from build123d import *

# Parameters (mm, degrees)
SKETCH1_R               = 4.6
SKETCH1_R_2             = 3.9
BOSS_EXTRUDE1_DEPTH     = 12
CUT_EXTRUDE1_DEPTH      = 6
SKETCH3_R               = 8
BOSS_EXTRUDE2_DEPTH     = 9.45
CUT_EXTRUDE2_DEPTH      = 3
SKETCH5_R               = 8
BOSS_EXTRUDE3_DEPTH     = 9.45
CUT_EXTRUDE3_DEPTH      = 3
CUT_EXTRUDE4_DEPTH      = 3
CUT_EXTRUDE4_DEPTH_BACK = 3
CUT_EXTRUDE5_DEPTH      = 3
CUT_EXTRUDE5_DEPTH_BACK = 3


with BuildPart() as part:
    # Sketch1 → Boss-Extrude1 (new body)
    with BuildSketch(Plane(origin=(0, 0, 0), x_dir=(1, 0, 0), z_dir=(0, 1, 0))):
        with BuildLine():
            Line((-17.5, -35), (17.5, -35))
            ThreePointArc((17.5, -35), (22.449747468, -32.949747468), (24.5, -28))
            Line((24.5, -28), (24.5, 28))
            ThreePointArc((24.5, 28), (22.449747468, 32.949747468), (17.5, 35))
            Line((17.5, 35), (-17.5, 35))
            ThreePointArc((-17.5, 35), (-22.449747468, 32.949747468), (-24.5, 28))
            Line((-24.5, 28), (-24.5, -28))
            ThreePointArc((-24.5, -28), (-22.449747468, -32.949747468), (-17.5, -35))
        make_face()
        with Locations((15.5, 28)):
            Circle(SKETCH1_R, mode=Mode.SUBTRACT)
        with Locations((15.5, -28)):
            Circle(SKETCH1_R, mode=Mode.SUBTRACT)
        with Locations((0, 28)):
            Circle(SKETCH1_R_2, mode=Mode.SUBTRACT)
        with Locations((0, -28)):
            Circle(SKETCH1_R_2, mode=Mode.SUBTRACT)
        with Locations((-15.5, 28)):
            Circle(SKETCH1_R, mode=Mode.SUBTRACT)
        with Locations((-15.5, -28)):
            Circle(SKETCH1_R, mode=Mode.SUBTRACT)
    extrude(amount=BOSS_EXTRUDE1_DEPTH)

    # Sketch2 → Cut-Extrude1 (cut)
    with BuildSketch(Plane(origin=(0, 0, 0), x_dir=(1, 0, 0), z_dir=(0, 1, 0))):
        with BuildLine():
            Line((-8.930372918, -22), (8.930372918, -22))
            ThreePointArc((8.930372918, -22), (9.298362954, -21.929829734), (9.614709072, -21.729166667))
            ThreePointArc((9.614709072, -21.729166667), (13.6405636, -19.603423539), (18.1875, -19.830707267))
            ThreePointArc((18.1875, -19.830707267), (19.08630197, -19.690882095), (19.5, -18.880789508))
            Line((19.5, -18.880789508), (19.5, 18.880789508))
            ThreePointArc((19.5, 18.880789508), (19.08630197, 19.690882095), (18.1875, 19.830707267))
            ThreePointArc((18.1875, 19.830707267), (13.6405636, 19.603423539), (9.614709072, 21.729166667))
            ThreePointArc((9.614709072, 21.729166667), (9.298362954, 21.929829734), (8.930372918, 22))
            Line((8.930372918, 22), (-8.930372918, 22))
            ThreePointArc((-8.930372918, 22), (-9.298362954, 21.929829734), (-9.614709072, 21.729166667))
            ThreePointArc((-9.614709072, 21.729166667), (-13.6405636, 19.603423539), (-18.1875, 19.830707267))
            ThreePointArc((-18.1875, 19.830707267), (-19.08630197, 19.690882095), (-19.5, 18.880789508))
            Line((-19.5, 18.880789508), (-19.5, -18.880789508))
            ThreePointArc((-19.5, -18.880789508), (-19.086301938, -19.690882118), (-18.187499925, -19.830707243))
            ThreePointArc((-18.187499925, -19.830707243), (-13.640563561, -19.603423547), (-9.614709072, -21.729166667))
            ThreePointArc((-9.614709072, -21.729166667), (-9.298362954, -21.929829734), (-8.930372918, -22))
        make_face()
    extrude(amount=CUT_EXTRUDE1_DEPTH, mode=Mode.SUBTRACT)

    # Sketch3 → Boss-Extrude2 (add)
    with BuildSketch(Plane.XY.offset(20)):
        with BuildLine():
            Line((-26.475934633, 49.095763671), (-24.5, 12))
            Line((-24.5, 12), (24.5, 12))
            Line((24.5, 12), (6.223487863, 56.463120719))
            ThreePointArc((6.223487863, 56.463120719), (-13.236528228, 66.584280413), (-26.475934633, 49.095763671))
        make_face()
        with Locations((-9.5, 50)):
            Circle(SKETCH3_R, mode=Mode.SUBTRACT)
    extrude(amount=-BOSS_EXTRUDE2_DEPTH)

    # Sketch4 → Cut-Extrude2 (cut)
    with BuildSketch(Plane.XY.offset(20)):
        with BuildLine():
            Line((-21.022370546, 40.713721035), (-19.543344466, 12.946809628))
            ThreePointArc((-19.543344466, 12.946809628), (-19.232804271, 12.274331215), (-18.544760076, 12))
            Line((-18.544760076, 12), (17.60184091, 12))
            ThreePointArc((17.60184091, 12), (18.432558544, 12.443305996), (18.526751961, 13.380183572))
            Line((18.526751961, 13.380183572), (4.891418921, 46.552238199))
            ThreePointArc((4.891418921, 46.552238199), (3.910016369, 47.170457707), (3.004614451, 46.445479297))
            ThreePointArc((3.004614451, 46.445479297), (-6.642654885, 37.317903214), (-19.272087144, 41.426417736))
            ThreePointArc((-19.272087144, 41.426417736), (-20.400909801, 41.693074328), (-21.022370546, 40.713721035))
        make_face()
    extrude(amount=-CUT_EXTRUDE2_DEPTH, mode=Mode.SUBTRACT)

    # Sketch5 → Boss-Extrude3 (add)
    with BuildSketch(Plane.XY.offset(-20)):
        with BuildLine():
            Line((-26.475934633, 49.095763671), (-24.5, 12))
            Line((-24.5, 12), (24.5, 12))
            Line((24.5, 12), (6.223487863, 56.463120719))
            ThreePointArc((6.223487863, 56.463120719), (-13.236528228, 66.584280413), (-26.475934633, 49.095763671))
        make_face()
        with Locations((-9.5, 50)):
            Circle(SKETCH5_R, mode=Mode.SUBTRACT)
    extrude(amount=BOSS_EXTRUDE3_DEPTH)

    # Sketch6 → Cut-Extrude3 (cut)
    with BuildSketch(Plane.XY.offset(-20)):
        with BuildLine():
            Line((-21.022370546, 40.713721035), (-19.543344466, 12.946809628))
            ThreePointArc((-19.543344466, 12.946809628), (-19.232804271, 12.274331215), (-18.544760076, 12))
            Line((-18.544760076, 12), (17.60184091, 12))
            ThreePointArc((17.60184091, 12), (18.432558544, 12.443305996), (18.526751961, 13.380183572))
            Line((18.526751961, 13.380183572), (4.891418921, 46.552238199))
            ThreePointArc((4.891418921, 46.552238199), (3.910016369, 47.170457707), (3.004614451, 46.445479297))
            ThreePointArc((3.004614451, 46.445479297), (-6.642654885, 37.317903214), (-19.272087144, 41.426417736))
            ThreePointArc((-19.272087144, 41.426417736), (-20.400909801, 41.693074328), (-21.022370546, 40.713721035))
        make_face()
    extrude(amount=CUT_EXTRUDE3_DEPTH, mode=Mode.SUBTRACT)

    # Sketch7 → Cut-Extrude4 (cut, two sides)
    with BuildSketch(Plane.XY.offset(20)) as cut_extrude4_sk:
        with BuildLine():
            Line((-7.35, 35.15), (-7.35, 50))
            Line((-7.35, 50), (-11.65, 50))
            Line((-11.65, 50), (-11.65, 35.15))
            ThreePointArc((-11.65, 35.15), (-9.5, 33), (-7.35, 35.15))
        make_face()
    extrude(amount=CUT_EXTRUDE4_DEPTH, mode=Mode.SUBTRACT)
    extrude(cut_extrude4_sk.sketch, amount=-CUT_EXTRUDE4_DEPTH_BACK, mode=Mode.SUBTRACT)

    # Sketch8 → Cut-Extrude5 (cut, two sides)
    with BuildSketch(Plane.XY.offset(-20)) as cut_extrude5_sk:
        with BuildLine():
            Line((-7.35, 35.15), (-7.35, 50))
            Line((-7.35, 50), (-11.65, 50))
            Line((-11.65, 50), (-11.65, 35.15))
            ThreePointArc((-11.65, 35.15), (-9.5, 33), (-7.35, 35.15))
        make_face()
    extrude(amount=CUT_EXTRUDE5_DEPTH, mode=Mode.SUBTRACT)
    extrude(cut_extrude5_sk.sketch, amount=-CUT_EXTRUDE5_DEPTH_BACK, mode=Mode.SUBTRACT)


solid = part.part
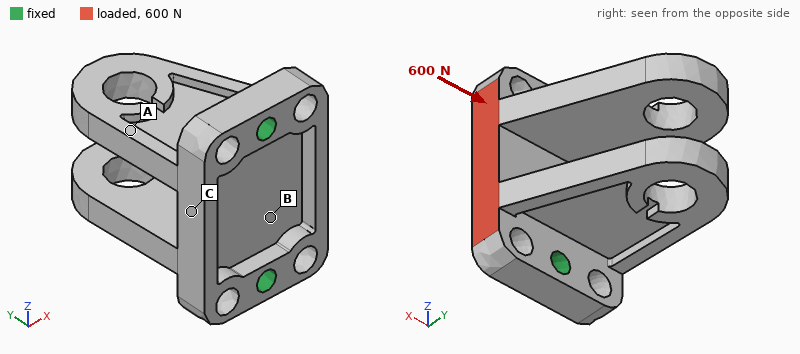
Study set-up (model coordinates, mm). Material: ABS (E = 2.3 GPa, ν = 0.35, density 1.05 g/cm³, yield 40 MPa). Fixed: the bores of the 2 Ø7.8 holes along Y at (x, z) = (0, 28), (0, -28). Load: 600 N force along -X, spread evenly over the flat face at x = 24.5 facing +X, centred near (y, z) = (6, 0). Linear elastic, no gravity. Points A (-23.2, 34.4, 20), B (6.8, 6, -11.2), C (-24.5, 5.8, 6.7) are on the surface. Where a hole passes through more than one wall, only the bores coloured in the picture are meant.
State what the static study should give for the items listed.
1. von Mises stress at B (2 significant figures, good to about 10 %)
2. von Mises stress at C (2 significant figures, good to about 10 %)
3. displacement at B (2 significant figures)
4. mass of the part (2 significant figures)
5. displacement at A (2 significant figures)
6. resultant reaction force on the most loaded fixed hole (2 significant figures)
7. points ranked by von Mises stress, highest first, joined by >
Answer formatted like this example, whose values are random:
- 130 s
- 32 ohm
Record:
- 1.6 MPa
- 0.81 MPa
- 21 µm
- 59 g
- 20 µm
- 310 N
- B > C > A
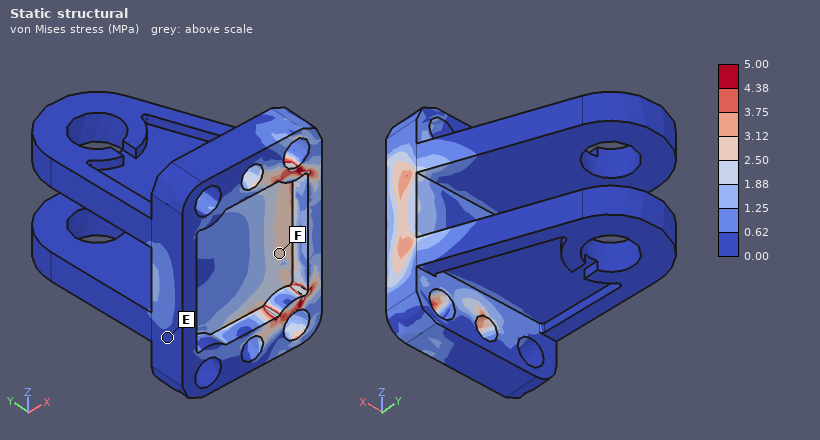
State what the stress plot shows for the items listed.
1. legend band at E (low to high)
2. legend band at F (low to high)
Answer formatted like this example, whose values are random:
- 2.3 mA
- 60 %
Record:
- 0.00 to 0.62 MPa
- 2.50 to 3.12 MPa
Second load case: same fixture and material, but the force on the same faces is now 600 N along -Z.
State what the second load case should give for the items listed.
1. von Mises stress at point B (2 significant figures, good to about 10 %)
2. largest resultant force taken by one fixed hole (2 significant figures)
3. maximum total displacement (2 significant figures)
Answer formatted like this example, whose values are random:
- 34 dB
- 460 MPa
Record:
- 2.8 MPa
- 380 N
- 73 µm
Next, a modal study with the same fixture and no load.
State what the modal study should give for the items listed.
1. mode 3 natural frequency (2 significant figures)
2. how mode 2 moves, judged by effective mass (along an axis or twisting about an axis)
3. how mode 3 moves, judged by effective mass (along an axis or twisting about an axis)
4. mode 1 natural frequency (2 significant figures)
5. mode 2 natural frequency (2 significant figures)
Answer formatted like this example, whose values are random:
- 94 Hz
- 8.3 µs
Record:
- 900 Hz
- along Z
- along X
- 570 Hz
- 640 Hz
